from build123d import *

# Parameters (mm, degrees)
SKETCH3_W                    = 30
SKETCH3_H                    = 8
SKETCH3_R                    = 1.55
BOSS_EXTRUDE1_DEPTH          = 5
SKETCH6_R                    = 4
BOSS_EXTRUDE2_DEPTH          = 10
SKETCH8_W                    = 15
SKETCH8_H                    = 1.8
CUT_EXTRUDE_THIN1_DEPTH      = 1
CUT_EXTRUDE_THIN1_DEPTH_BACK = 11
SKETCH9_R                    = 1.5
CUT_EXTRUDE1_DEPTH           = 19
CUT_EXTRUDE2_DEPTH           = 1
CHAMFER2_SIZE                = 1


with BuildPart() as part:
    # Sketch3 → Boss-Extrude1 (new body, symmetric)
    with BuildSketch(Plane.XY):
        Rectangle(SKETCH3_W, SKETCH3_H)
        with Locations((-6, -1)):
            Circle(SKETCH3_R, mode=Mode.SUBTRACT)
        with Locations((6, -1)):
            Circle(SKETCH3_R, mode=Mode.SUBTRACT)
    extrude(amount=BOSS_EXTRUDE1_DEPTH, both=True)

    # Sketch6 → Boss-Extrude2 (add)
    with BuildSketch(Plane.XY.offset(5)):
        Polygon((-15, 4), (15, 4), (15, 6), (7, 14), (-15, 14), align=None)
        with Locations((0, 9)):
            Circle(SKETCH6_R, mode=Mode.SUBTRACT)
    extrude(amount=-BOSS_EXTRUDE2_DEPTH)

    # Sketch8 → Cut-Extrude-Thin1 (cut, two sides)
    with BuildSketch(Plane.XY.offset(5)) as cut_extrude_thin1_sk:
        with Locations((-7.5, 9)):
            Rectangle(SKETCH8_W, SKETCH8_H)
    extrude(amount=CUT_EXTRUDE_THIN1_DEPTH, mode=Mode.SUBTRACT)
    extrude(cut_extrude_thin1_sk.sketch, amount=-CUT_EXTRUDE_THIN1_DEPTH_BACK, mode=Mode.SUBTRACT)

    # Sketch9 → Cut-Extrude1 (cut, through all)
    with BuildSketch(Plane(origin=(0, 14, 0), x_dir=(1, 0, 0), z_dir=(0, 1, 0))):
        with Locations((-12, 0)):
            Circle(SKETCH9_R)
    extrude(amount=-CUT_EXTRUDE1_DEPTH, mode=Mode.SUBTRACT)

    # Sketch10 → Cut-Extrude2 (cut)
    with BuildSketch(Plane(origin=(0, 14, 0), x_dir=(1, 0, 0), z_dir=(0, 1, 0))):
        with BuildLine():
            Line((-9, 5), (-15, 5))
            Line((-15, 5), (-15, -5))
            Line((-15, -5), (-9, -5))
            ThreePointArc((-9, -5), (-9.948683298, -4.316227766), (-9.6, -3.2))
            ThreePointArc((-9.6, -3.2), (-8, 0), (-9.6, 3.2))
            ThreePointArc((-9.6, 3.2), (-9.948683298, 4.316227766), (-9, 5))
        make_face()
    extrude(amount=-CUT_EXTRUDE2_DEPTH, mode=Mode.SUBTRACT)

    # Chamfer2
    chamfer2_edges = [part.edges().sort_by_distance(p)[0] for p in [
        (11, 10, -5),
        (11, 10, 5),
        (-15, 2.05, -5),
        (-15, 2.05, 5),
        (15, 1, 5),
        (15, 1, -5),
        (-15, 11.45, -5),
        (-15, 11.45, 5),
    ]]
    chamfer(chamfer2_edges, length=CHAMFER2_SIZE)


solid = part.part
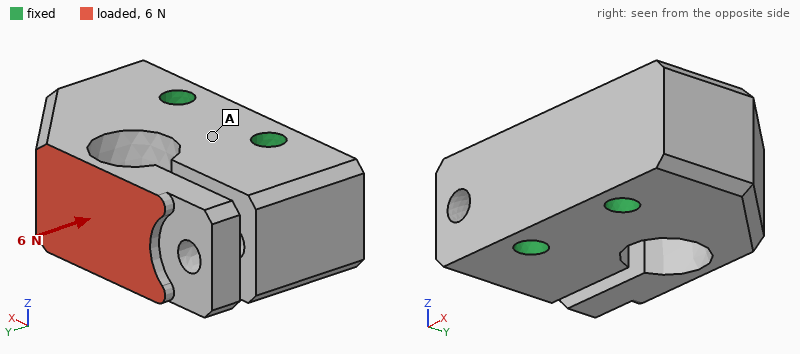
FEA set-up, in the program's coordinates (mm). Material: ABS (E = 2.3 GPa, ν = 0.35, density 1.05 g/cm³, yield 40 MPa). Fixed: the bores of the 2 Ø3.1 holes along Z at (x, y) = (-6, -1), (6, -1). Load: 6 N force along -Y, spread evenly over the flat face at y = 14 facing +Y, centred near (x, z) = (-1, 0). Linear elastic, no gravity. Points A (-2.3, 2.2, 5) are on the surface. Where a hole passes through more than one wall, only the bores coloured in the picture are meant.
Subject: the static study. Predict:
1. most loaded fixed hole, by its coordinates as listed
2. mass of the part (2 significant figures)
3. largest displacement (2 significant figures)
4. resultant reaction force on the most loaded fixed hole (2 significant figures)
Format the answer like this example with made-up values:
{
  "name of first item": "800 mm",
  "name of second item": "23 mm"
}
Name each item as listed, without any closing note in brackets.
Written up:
{
  "most loaded fixed hole, by its coordinates as listed": "(6, -1)",
  "mass of the part": "4.2 g",
  "largest displacement": "0.43 mm",
  "resultant reaction force on the most loaded fixed hole": "4.3 N"
}
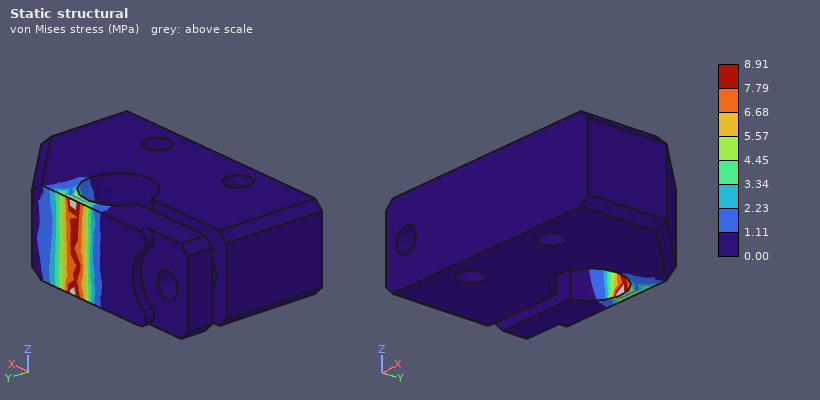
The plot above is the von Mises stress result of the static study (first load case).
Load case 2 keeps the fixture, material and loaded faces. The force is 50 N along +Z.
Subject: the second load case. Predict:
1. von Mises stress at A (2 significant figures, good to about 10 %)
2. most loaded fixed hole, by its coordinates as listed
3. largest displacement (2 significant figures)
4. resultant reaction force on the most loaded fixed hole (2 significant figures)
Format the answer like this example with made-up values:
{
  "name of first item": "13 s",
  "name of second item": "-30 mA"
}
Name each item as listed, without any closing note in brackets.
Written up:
{
  "von Mises stress at A": "0.99 MPa",
  "most loaded fixed hole, by its coordinates as listed": "(6, -1)",
  "largest displacement": "0.29 mm",
  "resultant reaction force on the most loaded fixed hole": "33 N"
}
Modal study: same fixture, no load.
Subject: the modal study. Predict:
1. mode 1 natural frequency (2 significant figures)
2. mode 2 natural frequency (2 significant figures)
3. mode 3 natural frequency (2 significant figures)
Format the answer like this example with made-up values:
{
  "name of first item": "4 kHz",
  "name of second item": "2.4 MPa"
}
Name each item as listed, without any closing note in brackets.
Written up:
{
  "mode 1 natural frequency": "630 Hz",
  "mode 2 natural frequency": "2200 Hz",
  "mode 3 natural frequency": "3800 Hz"
}
